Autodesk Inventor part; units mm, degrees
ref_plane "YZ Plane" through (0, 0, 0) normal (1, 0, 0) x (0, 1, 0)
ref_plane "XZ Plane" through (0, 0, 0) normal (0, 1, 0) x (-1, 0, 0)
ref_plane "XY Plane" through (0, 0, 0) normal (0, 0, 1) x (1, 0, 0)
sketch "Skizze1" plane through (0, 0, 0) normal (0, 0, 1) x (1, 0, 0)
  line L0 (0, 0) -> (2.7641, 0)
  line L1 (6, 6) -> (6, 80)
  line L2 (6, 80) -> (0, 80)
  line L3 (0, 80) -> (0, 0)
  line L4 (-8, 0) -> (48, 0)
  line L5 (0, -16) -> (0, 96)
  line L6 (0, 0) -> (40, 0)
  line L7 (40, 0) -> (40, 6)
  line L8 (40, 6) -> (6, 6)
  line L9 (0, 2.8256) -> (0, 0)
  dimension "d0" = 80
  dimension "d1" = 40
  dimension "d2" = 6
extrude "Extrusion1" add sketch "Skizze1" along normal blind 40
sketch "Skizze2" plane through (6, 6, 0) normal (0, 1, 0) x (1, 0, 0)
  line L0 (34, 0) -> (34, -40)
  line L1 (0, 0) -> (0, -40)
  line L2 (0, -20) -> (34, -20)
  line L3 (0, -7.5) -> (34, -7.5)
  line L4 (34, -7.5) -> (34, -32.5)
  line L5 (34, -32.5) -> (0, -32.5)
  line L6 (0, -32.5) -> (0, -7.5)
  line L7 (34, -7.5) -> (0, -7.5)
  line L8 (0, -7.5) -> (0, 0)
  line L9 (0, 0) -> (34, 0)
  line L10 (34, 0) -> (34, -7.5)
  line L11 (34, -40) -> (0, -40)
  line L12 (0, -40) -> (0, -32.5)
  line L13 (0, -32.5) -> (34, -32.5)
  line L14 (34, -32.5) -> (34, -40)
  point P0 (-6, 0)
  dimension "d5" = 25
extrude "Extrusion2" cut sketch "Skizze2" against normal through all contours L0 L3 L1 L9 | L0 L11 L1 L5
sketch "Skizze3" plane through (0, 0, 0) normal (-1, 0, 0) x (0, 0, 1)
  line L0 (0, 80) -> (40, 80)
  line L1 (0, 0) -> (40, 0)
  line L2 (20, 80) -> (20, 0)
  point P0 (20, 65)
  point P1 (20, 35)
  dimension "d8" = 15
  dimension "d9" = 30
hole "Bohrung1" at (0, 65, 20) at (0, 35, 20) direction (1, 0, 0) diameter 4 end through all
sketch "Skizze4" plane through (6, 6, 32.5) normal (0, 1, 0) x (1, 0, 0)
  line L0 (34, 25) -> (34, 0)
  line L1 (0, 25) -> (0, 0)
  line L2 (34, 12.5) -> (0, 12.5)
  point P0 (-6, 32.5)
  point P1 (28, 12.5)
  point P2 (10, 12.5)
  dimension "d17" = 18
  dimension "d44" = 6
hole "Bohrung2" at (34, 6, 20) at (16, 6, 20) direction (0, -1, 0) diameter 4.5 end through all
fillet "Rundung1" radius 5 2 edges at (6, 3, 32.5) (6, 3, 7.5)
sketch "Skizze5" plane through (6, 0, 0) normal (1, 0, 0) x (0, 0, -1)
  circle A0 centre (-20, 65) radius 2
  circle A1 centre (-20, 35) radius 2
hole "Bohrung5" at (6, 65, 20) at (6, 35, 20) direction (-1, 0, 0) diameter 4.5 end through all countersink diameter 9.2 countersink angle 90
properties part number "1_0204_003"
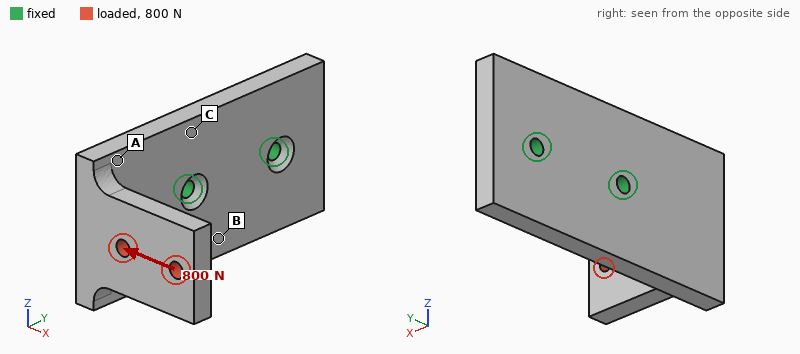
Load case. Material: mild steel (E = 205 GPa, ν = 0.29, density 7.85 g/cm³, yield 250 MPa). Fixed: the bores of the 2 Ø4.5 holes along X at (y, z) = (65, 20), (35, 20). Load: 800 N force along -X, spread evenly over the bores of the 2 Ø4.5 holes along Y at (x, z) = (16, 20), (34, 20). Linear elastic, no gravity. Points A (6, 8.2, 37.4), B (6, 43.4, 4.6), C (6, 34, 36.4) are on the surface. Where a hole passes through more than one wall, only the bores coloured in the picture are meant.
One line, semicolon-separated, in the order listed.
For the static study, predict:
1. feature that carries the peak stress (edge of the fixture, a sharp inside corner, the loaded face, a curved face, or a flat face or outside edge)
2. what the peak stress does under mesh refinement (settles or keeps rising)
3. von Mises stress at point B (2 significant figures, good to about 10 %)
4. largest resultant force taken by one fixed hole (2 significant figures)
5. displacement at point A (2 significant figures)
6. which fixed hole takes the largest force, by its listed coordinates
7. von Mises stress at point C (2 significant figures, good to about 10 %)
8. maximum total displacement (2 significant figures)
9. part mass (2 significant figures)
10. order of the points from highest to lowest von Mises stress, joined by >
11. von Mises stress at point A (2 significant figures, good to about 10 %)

edge of the fixture; keeps rising; 43 MPa; 1.5 kN; 0.070 mm; (35, 20); 72 MPa; 0.17 mm; 190 g; C > B > A; 18 MPa
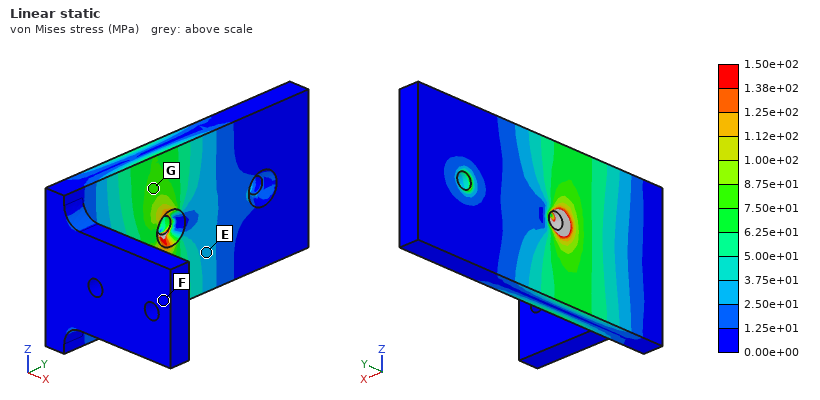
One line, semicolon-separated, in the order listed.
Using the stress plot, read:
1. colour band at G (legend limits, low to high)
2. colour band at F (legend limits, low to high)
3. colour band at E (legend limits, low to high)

7.50e+01 to 8.75e+01 MPa; 0.00e+00 to 1.25e+01 MPa; 2.50e+01 to 3.75e+01 MPa
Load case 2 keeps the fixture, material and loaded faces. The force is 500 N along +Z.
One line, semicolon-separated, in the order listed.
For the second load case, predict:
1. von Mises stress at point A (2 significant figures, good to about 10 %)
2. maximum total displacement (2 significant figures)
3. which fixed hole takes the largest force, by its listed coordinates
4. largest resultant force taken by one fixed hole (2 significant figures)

27 MPa; 89 µm; (35, 20); 950 N
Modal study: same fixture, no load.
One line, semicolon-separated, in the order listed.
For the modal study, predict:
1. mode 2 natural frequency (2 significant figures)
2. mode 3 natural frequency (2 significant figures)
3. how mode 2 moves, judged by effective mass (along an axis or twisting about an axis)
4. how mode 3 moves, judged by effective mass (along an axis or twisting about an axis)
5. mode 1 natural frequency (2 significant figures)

2200 Hz; 3800 Hz; along Z; along X; 1500 Hz
